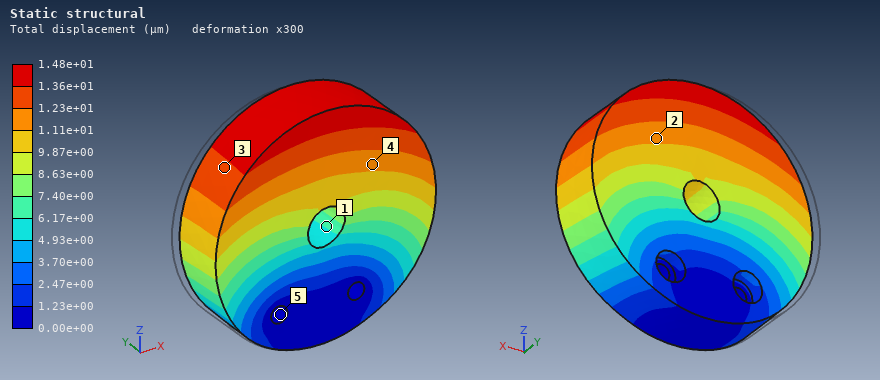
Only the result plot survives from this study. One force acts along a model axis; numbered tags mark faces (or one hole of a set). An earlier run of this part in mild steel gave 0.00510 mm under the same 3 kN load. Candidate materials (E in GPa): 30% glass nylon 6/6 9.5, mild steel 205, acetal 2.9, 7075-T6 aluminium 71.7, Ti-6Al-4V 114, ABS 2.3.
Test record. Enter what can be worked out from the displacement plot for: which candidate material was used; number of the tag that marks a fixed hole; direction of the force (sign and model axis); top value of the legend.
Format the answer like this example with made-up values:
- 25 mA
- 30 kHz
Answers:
- 7075-T6 aluminium
- 5
- +X
- 1.48e+01 µm
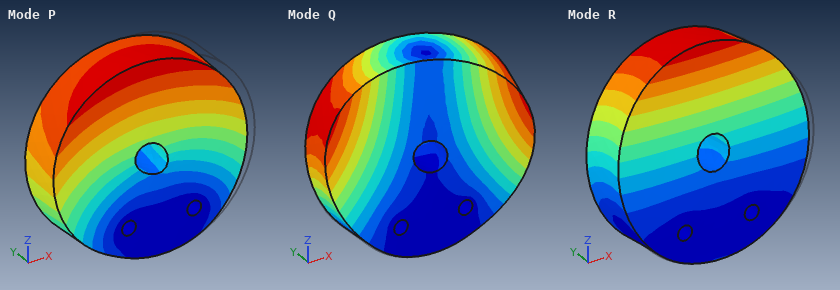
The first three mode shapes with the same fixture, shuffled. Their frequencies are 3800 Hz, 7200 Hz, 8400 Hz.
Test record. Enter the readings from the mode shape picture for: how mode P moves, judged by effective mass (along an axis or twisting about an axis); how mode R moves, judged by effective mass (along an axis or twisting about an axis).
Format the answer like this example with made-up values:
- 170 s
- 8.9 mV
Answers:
- along X
- along Y
